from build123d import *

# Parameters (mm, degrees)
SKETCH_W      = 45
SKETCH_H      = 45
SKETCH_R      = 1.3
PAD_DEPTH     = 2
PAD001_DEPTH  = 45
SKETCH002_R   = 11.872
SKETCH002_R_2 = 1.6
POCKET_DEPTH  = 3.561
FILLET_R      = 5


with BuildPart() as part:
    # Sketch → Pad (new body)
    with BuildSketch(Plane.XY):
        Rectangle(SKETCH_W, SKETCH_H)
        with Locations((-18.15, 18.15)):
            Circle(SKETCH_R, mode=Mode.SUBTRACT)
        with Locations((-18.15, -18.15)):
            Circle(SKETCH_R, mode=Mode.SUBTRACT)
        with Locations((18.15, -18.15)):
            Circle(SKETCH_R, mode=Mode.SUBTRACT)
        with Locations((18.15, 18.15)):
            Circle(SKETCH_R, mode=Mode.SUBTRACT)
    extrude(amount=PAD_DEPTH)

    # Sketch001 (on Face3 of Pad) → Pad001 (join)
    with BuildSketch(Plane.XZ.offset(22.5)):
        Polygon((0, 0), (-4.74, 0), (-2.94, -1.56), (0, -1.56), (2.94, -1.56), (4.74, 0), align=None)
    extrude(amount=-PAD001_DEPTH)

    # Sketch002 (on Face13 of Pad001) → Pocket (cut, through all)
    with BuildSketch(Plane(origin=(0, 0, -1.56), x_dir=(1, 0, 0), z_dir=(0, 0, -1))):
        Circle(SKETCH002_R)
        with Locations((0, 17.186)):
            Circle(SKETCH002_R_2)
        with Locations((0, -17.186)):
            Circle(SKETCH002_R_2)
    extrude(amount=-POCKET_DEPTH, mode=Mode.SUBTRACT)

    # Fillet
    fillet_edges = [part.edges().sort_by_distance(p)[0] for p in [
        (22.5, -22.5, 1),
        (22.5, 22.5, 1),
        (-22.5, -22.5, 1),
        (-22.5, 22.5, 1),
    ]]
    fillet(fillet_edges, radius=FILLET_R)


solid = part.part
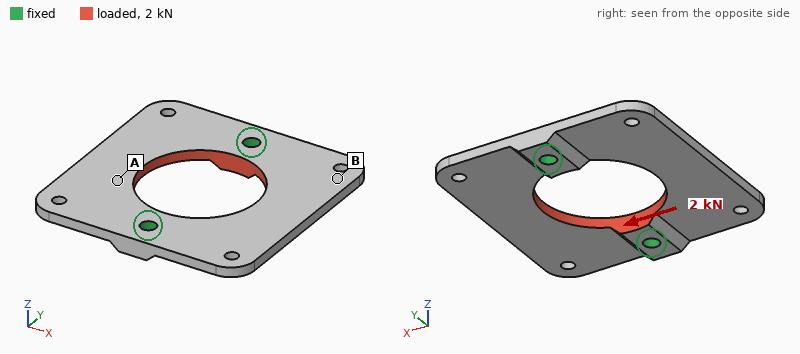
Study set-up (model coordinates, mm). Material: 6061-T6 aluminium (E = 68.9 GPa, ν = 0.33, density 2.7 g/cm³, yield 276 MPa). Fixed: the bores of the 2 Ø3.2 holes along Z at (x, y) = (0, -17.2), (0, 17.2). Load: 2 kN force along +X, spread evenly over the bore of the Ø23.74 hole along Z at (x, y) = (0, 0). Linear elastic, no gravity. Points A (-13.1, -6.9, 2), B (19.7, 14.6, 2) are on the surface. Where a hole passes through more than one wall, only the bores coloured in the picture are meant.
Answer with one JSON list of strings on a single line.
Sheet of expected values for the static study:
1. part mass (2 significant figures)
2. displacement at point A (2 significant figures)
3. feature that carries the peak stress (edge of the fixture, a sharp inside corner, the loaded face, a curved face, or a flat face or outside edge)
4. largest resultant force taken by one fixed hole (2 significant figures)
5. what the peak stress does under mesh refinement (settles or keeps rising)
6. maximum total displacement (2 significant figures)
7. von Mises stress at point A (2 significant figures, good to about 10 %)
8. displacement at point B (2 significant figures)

["8.9 g", "9.5 µm", "edge of the fixture", "1.0 kN", "keeps rising", "12 µm", "15 MPa", "8.1 µm"]
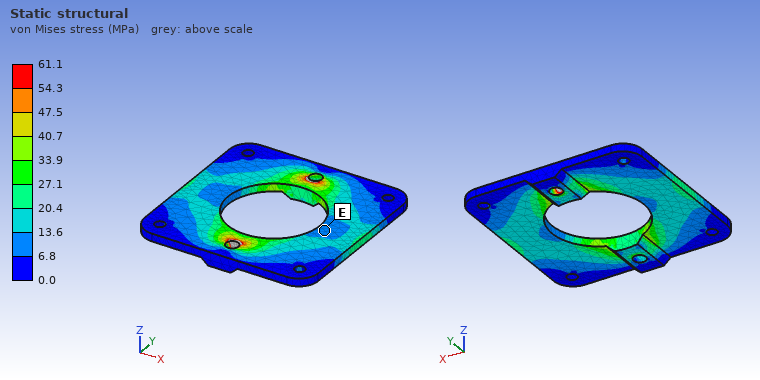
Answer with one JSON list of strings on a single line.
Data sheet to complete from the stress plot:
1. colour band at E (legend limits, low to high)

["6.8 to 13.6 MPa"]
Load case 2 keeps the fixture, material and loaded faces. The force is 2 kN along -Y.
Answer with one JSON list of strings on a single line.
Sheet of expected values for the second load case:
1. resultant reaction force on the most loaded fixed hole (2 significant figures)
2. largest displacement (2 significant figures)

["1.0 kN", "12 µm"]
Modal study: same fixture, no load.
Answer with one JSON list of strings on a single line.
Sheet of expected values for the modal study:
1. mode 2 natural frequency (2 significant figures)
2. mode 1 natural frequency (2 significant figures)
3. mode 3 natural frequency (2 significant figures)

["3200 Hz", "3100 Hz", "5900 Hz"]
